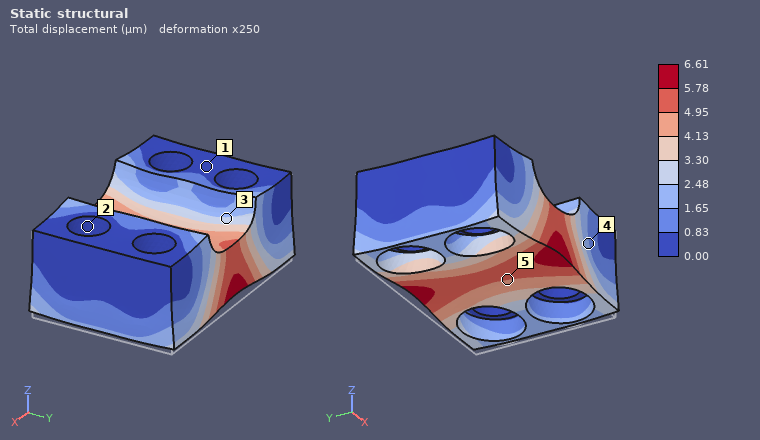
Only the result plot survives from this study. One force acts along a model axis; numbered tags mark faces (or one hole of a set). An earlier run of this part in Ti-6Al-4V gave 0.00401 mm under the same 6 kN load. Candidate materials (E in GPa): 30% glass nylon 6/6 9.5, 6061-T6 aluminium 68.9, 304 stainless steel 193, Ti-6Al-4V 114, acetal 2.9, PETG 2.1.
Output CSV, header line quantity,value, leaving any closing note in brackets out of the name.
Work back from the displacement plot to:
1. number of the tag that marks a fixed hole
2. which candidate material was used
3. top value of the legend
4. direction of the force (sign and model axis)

quantity,value
number of the tag that marks a fixed hole,2
which candidate material was used,6061-T6 aluminium
top value of the legend,6.61 µm
direction of the force,+Z
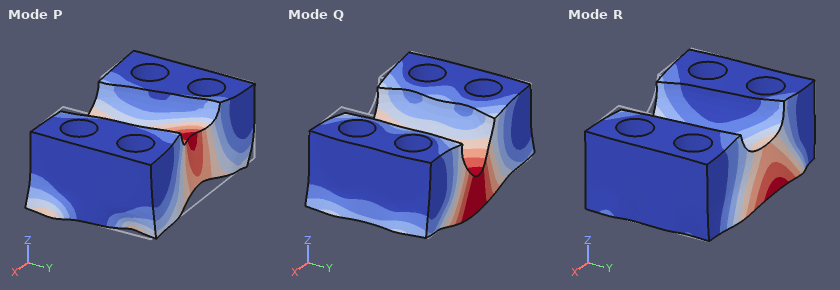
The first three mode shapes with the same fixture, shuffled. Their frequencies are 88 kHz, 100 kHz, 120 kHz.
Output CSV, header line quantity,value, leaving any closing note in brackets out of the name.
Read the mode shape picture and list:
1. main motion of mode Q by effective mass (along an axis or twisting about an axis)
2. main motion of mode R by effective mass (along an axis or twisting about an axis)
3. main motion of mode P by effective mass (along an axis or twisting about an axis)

quantity,value
main motion of mode Q by effective mass,along Z
main motion of mode R by effective mass,along Y
main motion of mode P by effective mass,along Y
